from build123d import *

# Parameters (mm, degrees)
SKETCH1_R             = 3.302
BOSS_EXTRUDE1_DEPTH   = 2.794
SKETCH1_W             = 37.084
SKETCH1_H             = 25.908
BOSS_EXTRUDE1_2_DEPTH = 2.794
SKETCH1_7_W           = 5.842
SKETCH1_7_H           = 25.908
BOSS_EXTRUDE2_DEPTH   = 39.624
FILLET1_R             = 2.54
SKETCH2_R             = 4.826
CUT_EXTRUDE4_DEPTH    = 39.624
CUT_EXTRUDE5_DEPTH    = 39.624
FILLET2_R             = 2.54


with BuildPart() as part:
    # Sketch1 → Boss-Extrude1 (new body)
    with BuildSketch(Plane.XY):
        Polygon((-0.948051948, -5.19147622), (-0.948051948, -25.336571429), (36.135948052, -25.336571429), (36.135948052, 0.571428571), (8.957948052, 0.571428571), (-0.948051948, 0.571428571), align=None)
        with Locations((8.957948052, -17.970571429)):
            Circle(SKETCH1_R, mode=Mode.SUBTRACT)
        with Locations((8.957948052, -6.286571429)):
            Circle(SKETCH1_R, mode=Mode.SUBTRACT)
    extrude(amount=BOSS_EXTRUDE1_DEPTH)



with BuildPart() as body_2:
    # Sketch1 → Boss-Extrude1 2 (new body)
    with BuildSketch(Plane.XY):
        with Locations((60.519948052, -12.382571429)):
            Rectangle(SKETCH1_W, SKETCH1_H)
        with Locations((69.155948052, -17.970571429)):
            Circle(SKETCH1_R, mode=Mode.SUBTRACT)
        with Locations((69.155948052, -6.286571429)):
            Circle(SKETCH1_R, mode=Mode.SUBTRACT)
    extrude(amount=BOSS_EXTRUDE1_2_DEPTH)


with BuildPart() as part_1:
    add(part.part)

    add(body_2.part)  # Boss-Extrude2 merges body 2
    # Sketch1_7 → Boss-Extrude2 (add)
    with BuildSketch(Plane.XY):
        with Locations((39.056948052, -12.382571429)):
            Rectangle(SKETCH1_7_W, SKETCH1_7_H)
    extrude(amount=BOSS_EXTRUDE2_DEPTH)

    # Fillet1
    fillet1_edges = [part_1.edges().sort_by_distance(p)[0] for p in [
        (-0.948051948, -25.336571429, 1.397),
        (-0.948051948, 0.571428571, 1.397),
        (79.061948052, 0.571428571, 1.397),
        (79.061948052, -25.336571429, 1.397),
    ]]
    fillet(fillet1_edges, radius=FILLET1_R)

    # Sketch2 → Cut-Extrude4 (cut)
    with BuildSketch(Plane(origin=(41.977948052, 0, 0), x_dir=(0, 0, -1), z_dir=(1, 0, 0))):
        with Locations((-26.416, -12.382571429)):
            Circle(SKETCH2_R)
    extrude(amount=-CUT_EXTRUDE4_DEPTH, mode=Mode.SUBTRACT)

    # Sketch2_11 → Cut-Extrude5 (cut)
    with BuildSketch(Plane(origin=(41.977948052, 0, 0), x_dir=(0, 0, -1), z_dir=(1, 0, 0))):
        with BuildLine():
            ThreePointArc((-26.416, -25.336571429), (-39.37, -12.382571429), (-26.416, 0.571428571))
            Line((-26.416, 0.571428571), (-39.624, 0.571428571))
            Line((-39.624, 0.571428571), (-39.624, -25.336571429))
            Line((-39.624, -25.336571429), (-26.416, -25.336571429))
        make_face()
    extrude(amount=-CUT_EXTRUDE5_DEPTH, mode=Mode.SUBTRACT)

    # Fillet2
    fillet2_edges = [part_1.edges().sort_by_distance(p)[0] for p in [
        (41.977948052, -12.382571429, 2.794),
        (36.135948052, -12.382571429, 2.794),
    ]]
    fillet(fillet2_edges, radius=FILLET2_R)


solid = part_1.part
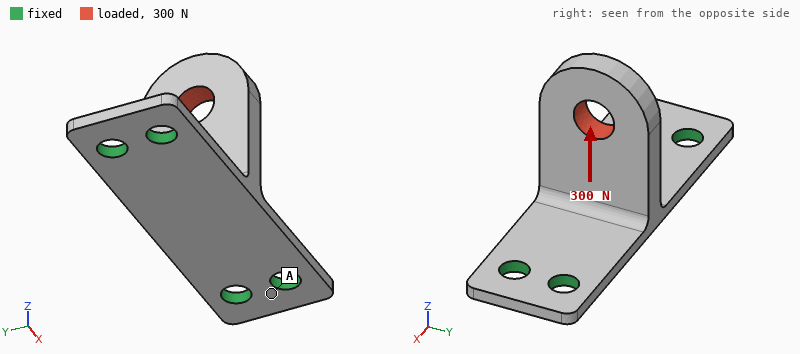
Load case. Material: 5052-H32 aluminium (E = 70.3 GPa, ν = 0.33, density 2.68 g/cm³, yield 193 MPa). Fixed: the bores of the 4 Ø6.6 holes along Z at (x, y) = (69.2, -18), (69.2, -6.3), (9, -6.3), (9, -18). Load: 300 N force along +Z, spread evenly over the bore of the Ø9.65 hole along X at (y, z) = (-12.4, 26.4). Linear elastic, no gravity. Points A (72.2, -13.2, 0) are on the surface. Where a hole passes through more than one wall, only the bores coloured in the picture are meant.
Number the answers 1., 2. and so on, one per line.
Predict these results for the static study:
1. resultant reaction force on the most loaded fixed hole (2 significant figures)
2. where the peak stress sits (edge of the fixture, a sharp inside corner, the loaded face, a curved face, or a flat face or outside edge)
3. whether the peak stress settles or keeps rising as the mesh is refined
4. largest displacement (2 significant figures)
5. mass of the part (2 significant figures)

1. 87 N
2. edge of the fixture
3. keeps rising
4. 57 µm
5. 27 g
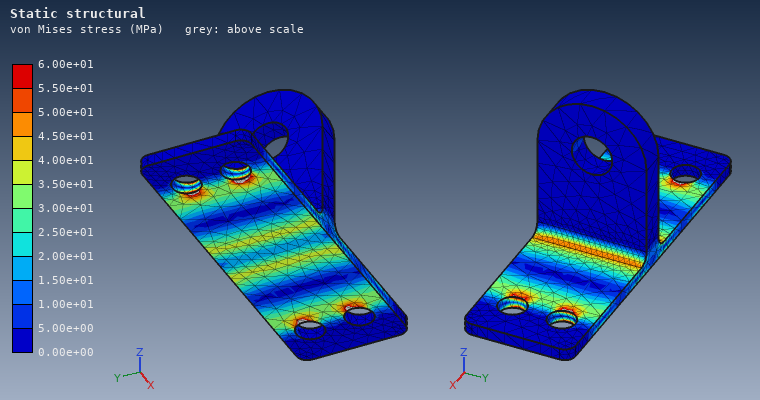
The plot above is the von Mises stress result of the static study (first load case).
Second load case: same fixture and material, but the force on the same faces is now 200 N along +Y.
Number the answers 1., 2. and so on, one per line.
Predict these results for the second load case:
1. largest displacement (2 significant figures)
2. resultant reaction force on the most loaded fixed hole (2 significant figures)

1. 0.29 mm
2. 190 N
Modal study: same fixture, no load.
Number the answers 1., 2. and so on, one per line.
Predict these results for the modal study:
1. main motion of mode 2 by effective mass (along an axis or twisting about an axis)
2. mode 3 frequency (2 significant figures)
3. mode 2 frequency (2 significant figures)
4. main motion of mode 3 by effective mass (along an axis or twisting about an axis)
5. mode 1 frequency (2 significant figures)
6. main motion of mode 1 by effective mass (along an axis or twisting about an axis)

1. along X
2. 2800 Hz
3. 2300 Hz
4. along Z
5. 1600 Hz
6. along Y
